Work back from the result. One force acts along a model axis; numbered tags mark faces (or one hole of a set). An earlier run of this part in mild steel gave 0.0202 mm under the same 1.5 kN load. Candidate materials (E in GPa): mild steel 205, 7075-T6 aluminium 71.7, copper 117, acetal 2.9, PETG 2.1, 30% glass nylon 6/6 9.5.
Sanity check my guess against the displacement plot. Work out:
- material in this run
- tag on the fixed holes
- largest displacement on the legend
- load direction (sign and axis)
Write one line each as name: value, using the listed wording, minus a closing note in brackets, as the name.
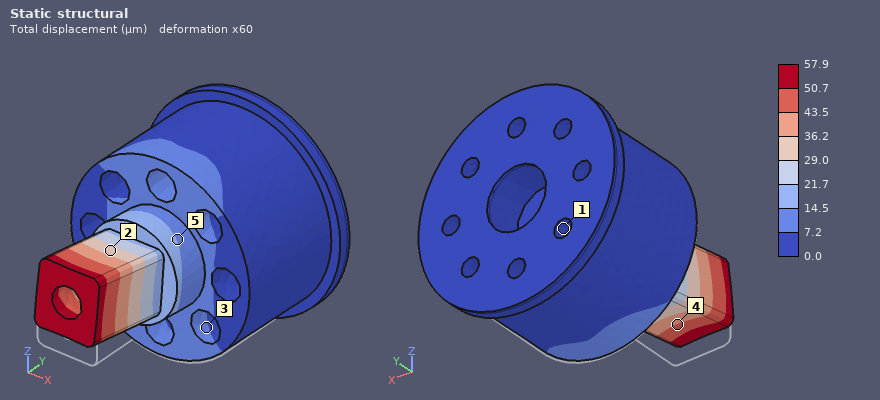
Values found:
material in this run: 7075-T6 aluminium
tag on the fixed holes: 1
largest displacement on the legend: 57.9 µm
load direction: +Z
